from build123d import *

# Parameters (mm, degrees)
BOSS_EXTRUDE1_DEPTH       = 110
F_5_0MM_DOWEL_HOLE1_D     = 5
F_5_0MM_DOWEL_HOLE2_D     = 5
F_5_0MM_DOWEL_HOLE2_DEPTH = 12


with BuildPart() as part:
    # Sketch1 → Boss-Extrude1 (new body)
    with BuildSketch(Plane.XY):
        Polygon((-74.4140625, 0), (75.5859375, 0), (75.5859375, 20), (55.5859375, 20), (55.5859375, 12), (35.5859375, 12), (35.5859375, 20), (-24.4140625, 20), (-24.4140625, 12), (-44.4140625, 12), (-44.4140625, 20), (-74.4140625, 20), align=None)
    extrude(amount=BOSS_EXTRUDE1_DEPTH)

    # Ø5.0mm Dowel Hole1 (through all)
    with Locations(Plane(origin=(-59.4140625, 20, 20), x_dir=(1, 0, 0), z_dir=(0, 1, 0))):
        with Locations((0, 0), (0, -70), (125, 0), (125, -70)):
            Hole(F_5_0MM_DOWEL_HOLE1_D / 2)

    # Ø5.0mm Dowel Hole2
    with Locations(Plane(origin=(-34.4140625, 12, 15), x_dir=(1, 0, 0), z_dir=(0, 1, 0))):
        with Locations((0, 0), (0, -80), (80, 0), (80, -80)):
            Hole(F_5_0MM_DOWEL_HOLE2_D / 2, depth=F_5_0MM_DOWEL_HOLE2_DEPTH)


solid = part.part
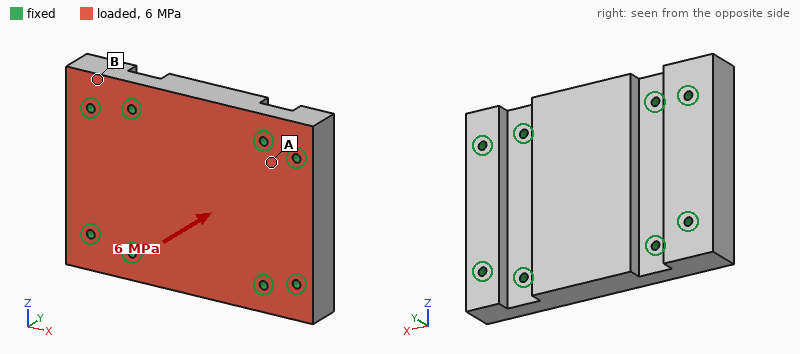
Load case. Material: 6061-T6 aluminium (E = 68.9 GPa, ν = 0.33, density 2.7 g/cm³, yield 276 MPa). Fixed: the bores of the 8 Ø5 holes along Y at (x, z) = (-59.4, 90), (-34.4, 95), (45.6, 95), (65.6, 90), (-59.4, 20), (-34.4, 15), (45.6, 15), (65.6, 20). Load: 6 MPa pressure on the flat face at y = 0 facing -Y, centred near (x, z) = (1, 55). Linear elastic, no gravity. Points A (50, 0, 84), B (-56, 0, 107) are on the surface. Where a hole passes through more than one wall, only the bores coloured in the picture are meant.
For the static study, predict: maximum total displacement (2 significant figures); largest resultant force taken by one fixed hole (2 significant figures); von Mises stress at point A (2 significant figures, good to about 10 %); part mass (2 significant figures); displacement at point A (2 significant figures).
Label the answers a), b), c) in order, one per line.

a) 87 µm
b) 16 kN
c) 46 MPa
d) 790 g
e) 21 µm
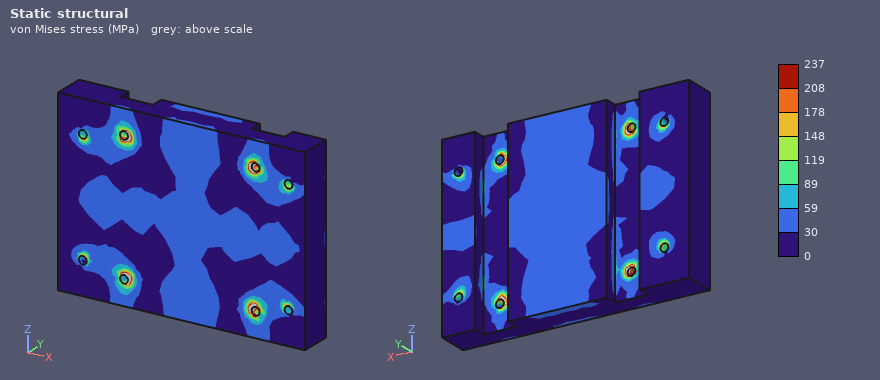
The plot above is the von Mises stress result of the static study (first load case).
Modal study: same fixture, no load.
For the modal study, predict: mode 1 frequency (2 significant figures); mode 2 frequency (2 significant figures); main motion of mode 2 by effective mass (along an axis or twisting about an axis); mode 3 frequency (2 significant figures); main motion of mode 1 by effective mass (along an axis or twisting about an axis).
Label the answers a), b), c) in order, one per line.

a) 6800 Hz
b) 9000 Hz
c) twisting about X
d) 11 kHz
e) along Y
